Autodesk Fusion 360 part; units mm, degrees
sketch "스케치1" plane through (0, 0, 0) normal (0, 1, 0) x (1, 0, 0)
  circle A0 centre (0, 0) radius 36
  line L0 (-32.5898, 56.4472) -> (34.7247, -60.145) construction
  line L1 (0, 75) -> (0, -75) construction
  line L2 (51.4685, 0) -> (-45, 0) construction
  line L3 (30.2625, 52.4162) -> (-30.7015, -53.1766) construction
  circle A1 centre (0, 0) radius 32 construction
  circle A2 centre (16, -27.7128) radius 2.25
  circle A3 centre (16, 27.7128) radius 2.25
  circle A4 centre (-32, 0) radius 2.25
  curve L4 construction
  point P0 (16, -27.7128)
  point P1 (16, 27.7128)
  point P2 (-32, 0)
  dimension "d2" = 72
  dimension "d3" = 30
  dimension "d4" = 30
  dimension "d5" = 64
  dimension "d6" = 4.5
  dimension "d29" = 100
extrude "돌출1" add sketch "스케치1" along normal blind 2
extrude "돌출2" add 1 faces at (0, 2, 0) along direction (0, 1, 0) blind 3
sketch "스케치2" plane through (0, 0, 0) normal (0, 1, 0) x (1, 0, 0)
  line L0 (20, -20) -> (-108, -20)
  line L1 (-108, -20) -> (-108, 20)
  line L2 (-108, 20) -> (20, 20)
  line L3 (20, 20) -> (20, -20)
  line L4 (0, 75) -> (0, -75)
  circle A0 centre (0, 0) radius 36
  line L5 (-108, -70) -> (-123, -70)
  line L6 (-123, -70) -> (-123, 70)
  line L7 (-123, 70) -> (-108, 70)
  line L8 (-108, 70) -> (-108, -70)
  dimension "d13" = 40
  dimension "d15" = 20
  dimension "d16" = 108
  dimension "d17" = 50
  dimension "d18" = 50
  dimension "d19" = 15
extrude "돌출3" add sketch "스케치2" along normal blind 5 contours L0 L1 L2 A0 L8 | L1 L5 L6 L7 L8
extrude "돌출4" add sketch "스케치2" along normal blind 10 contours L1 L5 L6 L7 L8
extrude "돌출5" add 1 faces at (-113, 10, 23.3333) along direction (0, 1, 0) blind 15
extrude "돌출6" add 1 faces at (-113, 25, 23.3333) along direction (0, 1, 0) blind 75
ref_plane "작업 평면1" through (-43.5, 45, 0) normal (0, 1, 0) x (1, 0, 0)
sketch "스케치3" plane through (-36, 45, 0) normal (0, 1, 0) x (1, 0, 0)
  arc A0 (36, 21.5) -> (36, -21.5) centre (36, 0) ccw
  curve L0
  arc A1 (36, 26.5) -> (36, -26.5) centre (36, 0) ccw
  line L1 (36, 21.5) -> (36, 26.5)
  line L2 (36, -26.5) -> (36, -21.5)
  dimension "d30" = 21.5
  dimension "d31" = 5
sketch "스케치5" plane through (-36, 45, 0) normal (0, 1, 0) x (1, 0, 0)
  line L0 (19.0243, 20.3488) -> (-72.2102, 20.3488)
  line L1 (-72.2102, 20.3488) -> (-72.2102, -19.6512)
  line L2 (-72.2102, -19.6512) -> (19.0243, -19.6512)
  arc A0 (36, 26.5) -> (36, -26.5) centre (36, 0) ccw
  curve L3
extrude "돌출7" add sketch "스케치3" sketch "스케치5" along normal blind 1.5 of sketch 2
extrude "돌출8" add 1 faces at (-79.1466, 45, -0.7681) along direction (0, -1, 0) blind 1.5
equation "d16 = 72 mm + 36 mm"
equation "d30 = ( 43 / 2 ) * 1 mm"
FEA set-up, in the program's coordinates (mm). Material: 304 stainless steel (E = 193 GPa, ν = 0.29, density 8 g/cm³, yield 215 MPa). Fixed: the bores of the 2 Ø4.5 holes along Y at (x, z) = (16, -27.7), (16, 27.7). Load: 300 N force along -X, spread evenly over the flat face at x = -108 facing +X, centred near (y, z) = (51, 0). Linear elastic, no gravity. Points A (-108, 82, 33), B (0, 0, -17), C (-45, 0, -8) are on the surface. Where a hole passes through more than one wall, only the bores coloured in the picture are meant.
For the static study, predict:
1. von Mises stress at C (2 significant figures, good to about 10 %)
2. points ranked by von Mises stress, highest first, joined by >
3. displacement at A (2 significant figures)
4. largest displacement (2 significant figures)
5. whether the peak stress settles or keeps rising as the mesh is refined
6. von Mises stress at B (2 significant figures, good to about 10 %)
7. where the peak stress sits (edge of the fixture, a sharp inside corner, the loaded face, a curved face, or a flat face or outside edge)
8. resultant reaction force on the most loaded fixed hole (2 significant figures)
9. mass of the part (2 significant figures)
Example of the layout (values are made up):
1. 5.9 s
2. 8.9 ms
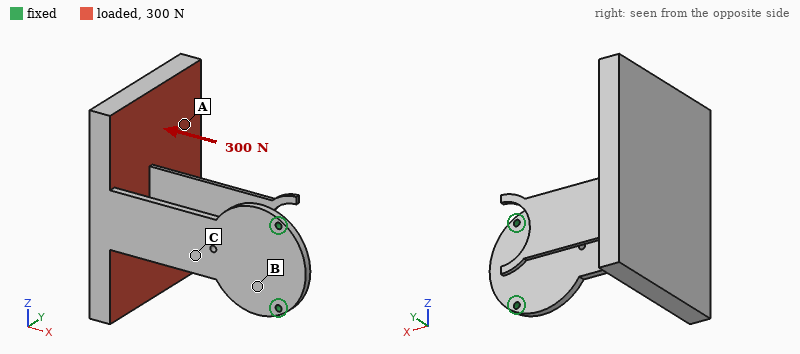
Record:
1. 85 MPa
2. C > B > A
3. 2.0 mm
4. 2.5 mm
5. keeps rising
6. 46 MPa
7. edge of the fixture
8. 150 N
9. 2.0 kg
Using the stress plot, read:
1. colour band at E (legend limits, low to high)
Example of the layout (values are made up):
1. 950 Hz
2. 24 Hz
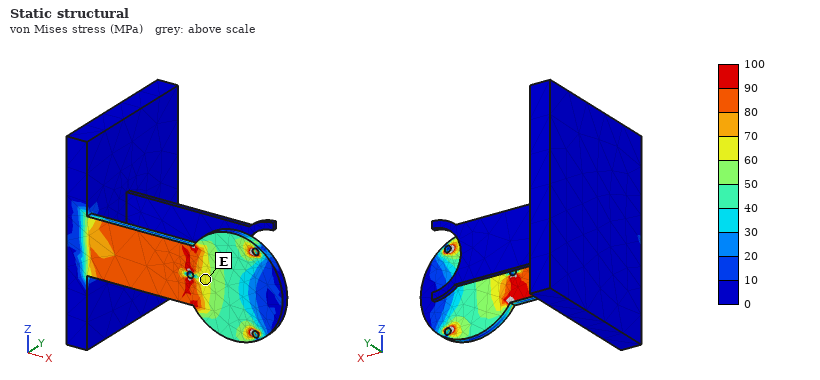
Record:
1. 60 to 70 MPa
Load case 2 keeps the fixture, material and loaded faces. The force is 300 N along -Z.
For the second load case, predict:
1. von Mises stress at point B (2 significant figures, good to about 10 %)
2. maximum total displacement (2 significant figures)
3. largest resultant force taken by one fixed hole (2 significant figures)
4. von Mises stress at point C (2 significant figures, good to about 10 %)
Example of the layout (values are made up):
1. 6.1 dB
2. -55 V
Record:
1. 34 MPa
2. 1.4 mm
3. 730 N
4. 75 MPa
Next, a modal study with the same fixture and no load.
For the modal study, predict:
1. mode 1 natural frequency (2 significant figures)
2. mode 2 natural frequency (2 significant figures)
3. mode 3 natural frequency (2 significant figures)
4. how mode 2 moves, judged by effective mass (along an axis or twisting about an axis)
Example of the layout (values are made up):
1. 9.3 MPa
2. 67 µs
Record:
1. 36 Hz
2. 62 Hz
3. 130 Hz
4. along Z
